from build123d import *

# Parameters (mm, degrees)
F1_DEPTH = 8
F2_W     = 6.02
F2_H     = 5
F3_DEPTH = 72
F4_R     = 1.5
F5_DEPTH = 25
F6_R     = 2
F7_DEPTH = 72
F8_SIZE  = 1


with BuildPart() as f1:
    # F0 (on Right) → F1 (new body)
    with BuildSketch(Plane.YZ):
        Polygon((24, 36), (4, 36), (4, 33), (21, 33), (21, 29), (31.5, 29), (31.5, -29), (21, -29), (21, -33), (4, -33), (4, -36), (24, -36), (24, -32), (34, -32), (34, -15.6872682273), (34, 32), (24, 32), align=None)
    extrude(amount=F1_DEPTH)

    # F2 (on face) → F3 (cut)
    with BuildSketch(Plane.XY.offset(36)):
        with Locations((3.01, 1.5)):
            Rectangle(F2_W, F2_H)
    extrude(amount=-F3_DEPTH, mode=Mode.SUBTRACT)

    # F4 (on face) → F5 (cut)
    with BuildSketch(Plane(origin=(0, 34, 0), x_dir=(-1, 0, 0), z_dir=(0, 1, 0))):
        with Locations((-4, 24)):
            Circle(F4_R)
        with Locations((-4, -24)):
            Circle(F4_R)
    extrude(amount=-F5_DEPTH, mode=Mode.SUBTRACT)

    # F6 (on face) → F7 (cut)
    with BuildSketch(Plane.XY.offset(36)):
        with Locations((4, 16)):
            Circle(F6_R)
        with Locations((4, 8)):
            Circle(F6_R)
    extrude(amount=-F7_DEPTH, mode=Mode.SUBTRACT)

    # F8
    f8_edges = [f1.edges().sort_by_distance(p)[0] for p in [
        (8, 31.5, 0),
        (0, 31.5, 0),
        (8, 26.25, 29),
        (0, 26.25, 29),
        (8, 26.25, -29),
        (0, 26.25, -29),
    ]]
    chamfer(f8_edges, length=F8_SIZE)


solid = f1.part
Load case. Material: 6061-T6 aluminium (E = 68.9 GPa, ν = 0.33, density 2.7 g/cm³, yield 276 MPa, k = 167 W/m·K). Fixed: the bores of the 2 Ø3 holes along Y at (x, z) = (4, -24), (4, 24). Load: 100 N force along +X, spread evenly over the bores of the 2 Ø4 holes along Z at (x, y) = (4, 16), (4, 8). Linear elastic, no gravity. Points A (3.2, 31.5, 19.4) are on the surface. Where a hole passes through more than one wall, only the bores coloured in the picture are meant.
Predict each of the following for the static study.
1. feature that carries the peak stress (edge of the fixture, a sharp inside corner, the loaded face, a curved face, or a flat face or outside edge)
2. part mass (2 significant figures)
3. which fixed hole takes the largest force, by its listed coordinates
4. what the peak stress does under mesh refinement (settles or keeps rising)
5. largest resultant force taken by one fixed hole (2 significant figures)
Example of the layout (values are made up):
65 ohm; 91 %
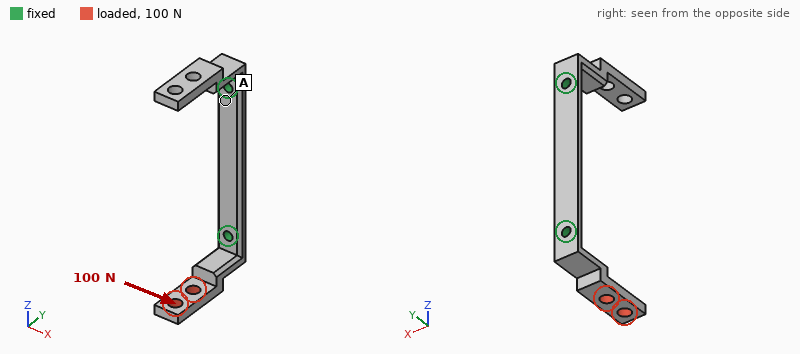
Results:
edge of the fixture; 6.8 g; (4, -24); keeps rising; 100 N
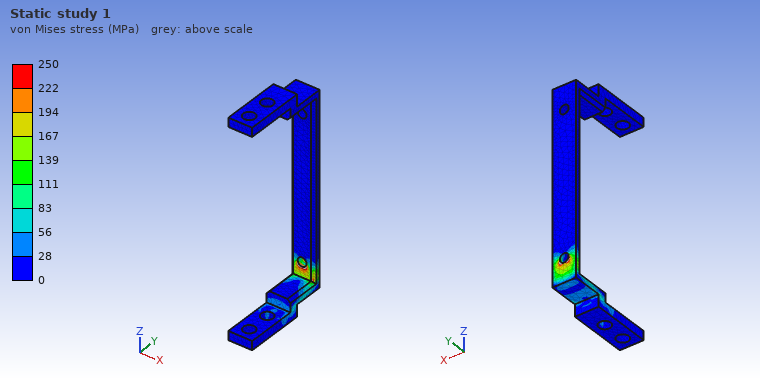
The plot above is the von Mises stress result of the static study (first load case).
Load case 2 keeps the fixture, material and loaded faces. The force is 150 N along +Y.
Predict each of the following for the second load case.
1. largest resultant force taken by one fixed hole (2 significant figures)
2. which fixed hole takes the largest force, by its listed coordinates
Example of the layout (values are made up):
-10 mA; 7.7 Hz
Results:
150 N; (4, -24)
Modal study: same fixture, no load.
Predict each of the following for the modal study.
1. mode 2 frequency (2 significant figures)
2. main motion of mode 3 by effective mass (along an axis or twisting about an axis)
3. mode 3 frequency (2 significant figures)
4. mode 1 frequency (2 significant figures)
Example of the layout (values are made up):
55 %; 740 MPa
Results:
2000 Hz; along X; 3100 Hz; 2000 Hz
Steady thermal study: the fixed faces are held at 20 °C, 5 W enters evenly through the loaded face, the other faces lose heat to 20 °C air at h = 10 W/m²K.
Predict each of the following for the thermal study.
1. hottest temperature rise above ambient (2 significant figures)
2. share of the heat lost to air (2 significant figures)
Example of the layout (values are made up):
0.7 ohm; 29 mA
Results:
40 K; 3.6 %
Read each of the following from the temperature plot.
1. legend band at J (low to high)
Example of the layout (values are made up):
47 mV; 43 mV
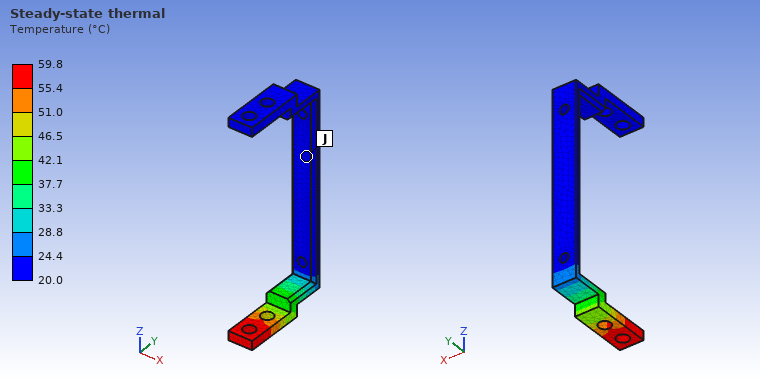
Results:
20.0 to 24.4 °C
